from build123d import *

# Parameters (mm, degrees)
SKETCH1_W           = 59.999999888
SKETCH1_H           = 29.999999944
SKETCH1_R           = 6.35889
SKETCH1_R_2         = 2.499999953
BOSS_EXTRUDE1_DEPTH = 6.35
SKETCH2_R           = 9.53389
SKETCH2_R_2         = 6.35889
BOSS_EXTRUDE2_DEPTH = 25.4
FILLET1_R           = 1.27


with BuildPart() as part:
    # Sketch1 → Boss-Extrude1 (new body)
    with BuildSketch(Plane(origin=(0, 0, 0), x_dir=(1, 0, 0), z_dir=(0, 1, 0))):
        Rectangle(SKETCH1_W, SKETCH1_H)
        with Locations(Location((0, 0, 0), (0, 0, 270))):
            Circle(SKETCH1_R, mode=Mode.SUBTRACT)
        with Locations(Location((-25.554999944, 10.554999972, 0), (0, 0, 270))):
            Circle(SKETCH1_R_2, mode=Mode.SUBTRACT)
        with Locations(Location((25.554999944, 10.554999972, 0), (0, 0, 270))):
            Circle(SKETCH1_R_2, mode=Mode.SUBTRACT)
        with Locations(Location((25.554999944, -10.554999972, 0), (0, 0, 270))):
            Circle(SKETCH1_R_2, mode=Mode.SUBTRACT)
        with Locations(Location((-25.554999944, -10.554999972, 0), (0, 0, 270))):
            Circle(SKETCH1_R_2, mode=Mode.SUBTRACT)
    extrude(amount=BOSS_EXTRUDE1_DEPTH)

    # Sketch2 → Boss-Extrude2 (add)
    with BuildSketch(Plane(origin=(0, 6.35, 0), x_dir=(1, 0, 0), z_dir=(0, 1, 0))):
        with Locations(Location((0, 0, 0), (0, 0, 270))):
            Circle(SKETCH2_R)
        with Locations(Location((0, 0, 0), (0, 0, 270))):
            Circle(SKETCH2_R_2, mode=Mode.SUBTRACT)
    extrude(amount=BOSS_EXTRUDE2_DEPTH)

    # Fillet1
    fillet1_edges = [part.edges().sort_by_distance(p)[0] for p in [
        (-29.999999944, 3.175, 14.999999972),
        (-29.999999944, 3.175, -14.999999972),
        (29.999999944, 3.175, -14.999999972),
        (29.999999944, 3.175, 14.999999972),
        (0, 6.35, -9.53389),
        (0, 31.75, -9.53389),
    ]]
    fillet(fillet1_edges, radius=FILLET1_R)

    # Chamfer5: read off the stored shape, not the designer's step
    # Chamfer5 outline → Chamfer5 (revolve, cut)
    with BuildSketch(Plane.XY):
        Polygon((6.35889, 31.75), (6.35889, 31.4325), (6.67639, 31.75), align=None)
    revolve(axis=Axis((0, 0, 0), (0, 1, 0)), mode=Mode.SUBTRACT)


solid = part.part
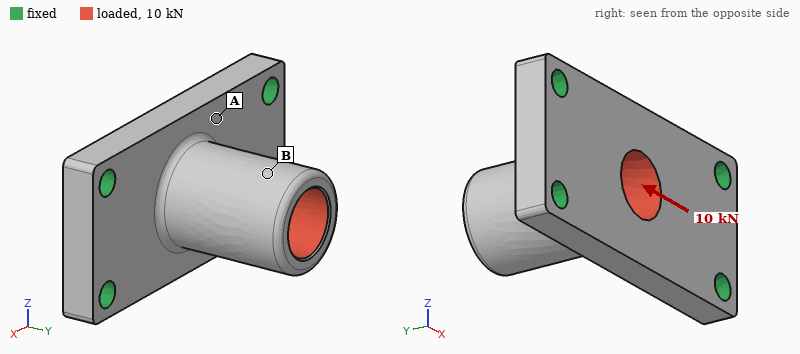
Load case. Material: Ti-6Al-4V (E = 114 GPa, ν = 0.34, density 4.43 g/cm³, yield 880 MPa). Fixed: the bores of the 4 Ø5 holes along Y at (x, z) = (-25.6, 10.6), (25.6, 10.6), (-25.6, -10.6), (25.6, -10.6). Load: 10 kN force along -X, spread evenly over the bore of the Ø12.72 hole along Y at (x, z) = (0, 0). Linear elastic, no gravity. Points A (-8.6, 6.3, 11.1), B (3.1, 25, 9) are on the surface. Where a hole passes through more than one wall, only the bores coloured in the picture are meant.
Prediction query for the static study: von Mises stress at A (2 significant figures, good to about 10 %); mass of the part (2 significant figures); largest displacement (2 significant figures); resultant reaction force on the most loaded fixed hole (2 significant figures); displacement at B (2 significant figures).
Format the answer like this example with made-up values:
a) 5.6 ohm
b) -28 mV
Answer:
a) 120 MPa
b) 63 g
c) 0.15 mm
d) 3.1 kN
e) 0.11 mm
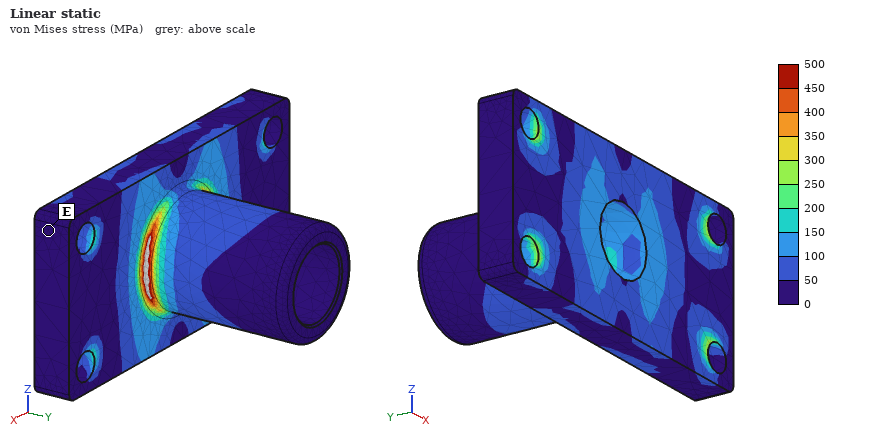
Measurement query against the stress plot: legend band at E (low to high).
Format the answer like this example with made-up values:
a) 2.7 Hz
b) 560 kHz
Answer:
a) 0 to 50 MPa
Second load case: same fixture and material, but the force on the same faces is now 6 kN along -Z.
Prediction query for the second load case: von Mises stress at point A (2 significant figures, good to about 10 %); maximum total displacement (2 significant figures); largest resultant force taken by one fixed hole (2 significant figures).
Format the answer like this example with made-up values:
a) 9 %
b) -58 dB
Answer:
a) 92 MPa
b) 0.17 mm
c) 2.8 kN
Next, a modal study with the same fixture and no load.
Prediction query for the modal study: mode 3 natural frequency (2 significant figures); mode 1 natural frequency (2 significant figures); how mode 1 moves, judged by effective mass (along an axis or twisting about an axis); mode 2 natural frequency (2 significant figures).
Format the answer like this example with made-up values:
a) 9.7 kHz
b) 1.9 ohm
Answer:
a) 10 kHz
b) 7100 Hz
c) along Z
d) 9900 Hz
